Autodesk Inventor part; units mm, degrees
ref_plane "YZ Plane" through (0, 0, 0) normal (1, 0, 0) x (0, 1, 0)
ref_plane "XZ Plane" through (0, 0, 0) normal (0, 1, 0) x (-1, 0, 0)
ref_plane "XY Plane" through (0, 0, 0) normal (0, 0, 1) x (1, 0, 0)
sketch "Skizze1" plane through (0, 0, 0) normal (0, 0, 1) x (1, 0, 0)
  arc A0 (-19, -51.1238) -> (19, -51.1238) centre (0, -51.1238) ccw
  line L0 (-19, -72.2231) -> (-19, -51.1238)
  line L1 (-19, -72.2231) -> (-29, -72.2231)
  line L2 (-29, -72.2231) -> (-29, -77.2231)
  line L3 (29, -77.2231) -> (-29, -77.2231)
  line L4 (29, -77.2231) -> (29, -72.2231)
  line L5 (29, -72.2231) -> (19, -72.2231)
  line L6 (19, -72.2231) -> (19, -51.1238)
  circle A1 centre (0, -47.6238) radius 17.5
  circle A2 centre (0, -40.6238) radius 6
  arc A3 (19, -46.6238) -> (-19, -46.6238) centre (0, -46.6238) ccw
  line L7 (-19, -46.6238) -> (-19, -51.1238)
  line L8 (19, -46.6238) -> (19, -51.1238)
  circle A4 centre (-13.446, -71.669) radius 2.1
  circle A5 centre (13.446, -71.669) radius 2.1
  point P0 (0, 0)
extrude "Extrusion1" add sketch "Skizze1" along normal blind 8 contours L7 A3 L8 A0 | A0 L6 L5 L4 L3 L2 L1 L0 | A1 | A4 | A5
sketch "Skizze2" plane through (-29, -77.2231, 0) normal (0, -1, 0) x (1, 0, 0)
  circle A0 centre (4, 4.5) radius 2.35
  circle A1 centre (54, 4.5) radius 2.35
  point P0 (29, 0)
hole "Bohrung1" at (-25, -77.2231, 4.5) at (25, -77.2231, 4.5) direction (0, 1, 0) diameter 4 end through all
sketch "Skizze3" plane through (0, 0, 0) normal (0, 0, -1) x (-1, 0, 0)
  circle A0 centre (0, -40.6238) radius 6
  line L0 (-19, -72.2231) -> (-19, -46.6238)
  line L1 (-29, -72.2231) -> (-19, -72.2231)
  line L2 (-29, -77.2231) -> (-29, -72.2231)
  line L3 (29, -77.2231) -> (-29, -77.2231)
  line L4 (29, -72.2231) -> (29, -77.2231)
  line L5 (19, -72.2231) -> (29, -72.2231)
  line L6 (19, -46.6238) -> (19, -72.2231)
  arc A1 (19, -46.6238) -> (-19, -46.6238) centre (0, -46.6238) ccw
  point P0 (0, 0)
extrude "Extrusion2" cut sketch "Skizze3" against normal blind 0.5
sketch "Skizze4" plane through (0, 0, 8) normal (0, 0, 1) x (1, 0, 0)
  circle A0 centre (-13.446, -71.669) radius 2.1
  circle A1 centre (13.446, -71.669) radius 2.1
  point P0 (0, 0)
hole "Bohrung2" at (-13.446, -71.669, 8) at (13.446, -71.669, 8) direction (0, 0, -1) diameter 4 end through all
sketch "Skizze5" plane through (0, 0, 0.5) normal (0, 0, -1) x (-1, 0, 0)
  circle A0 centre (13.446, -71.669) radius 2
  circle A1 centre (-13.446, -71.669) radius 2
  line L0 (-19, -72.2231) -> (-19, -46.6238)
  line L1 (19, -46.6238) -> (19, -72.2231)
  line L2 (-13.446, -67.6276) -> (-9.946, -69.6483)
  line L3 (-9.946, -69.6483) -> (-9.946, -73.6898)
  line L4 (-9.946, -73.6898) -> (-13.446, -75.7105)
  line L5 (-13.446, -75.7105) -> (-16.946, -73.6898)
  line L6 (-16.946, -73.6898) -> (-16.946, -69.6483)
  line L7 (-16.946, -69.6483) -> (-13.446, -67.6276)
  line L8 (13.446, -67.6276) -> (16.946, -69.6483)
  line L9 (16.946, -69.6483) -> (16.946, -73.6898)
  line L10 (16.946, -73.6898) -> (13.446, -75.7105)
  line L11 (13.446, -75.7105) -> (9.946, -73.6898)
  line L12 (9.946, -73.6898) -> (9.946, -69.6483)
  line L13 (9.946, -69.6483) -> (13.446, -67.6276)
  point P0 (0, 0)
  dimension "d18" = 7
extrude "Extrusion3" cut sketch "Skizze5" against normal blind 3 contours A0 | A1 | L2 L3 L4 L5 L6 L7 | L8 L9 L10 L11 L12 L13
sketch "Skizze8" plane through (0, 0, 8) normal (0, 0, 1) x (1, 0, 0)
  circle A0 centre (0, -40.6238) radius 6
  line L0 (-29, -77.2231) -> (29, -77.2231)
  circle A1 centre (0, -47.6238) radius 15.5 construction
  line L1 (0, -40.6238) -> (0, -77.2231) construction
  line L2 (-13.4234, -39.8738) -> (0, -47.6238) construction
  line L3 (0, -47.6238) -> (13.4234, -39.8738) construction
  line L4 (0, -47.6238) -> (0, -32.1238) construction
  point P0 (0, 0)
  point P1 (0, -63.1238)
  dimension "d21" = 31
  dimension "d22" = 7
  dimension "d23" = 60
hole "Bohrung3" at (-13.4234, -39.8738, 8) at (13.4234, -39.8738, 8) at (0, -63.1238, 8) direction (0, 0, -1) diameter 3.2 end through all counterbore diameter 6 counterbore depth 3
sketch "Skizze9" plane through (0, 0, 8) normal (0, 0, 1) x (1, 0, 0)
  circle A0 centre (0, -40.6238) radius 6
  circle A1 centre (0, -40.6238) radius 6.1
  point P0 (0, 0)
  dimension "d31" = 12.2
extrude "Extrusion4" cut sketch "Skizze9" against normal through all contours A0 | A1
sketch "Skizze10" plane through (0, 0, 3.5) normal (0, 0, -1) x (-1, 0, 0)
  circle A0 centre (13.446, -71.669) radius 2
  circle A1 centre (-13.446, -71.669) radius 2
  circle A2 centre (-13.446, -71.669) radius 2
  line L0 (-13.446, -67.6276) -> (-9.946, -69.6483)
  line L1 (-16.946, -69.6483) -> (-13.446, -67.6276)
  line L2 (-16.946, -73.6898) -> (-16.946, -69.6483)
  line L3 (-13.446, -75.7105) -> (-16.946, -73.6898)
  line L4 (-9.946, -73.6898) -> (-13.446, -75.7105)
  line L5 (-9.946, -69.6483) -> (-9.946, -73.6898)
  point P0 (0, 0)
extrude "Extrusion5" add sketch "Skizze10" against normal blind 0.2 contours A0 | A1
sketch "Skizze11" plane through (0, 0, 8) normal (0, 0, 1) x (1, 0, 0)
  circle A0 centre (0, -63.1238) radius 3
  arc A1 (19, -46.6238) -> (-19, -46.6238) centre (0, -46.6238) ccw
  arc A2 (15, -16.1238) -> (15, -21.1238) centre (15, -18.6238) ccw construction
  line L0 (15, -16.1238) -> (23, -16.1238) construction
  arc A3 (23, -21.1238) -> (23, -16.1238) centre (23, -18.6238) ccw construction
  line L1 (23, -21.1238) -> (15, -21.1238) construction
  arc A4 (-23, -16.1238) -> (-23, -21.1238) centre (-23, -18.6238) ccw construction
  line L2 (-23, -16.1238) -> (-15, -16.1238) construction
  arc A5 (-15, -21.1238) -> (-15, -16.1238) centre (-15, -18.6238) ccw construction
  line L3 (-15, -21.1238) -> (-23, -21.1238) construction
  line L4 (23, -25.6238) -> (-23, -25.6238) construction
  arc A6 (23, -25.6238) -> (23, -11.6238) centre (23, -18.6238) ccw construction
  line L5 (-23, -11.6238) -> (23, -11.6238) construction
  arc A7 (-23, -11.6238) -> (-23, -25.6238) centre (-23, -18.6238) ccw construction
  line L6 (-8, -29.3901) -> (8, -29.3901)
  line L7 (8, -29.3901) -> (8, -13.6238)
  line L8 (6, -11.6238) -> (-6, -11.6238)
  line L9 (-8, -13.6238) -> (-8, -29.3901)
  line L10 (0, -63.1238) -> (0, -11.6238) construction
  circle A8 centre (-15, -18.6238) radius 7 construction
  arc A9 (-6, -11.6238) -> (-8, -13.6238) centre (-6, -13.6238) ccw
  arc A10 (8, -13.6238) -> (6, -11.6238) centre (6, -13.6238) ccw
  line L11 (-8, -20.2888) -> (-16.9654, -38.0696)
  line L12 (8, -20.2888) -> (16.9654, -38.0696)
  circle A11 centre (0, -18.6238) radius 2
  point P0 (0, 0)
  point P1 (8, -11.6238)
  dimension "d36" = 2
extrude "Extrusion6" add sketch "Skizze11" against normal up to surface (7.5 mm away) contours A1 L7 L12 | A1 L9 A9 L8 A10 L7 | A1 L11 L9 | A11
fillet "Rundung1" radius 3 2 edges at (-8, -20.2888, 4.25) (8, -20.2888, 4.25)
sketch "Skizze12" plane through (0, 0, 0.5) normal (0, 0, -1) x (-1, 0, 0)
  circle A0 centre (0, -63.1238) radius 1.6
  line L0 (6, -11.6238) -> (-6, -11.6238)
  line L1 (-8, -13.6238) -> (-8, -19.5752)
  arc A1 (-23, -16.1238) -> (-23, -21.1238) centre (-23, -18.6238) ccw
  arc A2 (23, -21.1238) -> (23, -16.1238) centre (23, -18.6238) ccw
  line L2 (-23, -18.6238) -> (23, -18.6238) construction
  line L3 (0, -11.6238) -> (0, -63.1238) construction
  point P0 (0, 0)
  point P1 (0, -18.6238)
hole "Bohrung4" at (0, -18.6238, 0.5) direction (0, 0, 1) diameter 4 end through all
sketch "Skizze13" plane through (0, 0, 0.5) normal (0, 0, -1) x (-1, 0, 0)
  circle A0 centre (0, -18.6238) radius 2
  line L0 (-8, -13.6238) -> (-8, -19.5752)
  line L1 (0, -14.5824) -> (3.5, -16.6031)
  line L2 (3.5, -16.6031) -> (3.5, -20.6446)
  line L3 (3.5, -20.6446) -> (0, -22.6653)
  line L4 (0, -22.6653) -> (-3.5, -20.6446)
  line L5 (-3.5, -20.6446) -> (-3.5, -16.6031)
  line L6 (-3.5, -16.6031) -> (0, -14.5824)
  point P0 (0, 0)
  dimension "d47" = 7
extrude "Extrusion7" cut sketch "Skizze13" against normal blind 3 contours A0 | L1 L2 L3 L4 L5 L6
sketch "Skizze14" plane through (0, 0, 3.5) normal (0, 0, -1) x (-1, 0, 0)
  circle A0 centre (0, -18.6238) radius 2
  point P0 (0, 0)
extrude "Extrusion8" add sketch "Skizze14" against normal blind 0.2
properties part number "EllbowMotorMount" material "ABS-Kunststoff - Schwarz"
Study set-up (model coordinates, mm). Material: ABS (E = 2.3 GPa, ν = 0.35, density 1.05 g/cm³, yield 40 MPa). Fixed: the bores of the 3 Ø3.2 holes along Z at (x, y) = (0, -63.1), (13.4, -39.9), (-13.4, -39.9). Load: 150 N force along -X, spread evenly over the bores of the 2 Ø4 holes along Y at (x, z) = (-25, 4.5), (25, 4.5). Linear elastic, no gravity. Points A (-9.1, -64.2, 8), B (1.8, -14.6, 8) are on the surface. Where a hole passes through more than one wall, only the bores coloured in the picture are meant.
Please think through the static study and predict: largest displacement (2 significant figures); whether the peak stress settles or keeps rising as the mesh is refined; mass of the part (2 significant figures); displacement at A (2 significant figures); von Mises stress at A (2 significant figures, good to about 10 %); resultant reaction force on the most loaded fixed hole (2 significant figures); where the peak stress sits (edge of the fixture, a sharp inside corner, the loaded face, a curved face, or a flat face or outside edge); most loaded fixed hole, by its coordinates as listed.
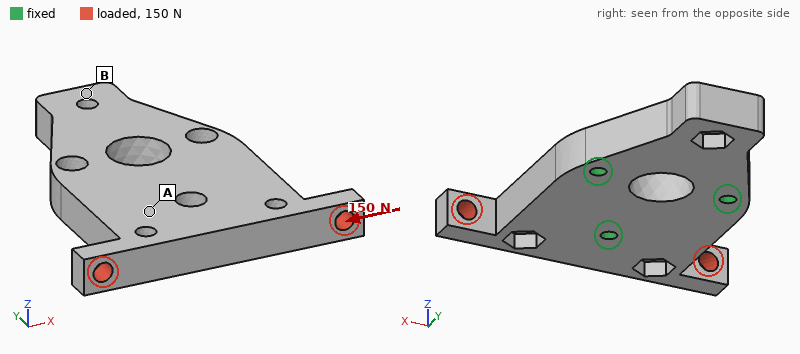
61 µm
keeps rising
15 g
12 µm
1.1 MPa
160 N
edge of the fixture
(0, -63.1)
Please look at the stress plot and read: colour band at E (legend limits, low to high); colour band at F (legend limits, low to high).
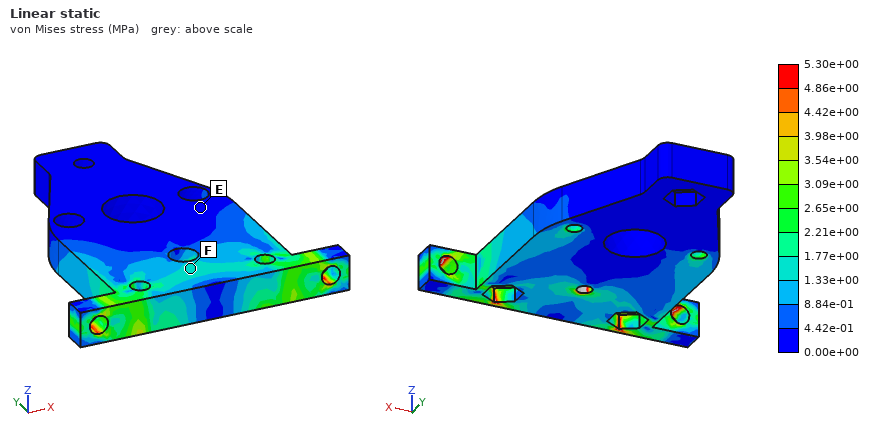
0.00e+00 to 4.42e-01 MPa
1.33e+00 to 1.77e+00 MPa
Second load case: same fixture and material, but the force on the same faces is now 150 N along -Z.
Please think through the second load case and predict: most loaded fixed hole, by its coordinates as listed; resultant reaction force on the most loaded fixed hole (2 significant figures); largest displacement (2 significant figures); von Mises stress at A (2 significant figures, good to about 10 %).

(0, -63.1)
200 N
0.66 mm
5.1 MPa
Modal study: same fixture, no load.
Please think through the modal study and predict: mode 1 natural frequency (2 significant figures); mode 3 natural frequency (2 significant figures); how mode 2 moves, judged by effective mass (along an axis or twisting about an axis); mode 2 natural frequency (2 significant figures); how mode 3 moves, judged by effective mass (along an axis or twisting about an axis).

1900 Hz
2900 Hz
twisting about Y
2200 Hz
along Z
